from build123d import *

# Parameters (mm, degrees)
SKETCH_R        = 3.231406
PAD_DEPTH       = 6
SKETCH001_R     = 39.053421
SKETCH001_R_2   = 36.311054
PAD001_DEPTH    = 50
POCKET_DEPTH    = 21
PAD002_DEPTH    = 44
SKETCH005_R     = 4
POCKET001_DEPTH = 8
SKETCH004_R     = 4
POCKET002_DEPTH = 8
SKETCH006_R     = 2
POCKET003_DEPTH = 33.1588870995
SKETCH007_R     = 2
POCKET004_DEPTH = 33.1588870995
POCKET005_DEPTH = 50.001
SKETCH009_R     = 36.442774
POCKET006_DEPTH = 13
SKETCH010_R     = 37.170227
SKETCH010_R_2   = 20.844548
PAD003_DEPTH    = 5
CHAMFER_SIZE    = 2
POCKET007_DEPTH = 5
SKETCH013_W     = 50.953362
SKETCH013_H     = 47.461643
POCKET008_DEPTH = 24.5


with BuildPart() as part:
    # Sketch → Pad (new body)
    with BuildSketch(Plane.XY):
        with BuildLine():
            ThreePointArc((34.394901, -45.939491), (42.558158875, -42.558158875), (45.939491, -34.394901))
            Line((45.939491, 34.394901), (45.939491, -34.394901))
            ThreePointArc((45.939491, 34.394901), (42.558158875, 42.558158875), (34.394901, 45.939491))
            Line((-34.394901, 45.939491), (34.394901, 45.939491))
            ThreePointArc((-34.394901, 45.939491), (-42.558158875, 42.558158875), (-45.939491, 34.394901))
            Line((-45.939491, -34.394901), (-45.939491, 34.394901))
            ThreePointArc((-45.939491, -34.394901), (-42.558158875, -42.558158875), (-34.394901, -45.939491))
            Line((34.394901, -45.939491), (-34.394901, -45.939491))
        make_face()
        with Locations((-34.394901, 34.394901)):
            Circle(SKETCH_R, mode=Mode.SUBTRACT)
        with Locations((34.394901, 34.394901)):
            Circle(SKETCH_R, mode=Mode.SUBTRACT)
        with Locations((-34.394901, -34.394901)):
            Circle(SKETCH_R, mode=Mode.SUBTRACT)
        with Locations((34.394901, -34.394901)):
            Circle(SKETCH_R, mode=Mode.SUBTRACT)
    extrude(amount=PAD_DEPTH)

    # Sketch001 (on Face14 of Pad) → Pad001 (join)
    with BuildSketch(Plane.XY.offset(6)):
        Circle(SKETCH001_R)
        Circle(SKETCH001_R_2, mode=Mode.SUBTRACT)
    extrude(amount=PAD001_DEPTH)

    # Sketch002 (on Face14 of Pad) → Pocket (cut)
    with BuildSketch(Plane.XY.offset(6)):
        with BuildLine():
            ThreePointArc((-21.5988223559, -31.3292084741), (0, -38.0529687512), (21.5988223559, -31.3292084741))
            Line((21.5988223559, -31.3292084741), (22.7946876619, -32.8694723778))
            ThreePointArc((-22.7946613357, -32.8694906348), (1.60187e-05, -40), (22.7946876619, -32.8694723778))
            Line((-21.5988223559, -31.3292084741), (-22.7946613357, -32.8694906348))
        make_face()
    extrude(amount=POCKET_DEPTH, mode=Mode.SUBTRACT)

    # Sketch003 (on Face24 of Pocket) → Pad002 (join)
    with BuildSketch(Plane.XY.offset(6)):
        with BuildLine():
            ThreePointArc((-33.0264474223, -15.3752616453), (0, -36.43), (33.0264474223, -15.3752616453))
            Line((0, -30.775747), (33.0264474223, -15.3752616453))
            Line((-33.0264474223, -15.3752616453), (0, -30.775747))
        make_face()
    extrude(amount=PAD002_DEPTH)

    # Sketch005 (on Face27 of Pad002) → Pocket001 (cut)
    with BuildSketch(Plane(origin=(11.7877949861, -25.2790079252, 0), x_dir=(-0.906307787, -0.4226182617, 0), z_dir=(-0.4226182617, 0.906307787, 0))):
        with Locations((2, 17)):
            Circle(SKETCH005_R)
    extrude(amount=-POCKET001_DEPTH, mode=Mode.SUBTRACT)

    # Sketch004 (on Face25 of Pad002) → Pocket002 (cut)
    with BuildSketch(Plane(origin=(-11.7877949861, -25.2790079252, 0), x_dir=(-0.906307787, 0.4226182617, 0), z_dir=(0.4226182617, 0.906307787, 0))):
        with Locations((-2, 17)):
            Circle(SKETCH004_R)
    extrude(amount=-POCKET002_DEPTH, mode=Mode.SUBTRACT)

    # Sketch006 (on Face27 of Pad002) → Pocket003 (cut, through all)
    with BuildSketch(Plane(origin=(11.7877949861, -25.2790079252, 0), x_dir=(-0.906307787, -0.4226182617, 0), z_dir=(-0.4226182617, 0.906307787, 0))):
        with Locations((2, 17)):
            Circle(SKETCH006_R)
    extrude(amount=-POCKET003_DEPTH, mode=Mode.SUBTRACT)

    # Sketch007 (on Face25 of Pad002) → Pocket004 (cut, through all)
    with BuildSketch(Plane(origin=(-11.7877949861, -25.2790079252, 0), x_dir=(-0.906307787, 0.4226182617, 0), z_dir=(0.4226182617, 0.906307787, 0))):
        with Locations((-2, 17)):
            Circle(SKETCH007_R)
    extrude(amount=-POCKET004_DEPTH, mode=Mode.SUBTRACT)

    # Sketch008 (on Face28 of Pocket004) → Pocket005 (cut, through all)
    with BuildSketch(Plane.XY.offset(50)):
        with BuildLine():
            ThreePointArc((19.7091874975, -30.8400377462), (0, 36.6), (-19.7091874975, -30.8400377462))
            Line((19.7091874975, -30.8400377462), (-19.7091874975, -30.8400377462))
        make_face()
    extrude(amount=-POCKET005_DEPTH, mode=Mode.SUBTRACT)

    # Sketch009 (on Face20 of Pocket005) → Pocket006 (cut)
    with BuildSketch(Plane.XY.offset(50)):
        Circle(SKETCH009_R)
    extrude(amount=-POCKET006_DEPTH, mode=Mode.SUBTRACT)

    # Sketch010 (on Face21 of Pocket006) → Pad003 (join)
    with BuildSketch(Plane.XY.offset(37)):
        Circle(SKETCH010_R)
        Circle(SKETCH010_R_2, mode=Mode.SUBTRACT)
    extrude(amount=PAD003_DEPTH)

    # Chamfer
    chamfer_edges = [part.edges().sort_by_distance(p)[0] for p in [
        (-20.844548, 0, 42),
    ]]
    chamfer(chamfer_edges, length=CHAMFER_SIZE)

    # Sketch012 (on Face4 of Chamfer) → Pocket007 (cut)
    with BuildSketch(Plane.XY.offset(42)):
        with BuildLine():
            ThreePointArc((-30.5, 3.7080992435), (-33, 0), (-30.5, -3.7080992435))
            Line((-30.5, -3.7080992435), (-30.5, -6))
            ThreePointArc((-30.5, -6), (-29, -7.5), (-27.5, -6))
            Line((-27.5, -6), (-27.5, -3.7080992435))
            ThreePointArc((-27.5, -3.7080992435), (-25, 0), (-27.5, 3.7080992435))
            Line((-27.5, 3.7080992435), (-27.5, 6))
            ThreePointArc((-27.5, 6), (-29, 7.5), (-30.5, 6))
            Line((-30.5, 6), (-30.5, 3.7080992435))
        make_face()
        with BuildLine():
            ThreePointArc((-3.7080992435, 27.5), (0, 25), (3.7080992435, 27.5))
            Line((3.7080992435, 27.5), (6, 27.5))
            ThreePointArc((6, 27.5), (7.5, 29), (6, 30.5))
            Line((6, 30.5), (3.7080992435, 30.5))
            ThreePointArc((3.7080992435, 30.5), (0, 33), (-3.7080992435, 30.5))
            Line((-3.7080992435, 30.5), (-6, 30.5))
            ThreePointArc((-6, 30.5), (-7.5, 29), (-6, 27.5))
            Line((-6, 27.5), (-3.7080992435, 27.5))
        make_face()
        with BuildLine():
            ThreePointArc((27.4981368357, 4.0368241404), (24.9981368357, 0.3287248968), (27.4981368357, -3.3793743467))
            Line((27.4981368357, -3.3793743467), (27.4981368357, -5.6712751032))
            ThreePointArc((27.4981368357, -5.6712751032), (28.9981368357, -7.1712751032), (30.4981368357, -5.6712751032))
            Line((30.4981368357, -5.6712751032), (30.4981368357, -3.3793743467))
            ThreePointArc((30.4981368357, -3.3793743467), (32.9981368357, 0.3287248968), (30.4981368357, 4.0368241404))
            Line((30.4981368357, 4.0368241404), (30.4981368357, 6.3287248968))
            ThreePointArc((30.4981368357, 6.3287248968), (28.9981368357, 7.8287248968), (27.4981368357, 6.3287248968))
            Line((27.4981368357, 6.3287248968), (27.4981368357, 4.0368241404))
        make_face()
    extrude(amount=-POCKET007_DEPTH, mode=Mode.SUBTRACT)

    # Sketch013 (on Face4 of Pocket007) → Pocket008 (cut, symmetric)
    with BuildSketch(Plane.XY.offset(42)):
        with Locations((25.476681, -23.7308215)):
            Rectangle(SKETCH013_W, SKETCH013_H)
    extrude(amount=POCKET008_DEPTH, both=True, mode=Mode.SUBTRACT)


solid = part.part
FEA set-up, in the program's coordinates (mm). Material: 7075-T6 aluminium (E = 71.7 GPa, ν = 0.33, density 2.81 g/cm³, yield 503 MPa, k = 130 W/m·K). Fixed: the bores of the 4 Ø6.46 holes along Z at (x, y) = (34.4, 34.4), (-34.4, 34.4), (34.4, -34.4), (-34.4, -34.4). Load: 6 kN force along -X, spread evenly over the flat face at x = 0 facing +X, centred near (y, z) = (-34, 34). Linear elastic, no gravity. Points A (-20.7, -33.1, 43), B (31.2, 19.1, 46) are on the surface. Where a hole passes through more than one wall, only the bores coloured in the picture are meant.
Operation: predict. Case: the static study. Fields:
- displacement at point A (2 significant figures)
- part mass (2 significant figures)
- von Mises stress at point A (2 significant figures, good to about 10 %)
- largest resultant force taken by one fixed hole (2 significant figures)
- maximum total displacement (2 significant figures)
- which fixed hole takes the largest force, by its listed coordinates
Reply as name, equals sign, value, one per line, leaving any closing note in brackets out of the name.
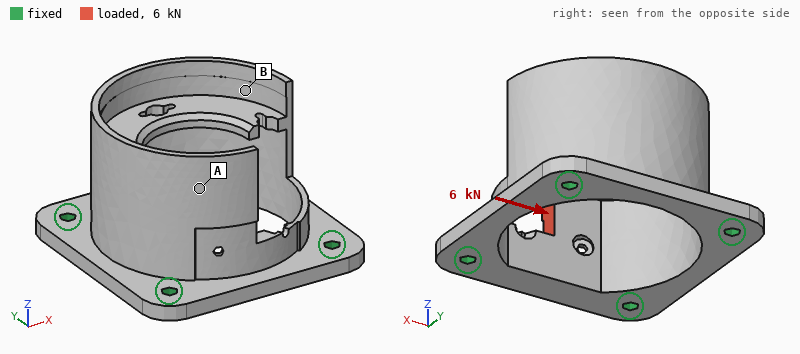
displacement at point A = 0.25 mm
part mass = 170 g
von Mises stress at point A = 54 MPa
largest resultant force taken by one fixed hole = 4.6 kN
maximum total displacement = 0.47 mm
which fixed hole takes the largest force, by its listed coordinates = (34.4, -34.4)
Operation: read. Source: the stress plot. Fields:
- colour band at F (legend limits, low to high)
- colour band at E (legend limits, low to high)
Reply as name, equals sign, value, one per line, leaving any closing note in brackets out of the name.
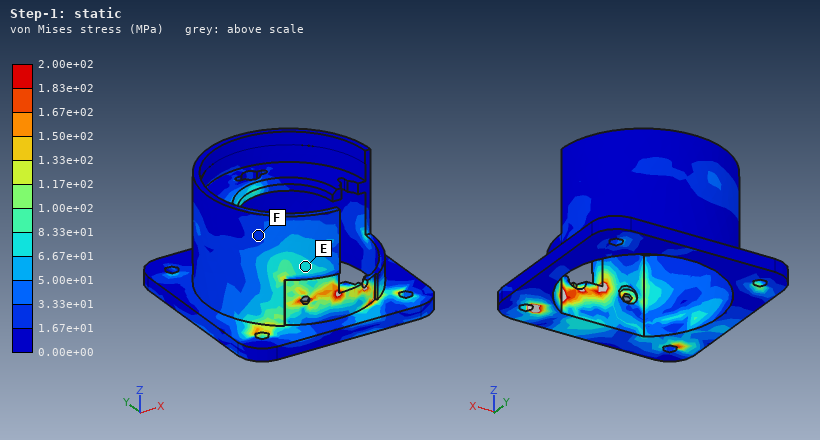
colour band at F = 1.67e+01 to 3.33e+01 MPa
colour band at E = 6.67e+01 to 8.33e+01 MPa
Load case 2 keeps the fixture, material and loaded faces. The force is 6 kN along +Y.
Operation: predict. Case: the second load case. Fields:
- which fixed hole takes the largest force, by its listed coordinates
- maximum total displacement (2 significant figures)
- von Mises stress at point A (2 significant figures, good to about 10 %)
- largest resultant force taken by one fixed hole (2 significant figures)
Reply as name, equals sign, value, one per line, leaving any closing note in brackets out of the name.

which fixed hole takes the largest force, by its listed coordinates = (-34.4, -34.4)
maximum total displacement = 1.0 mm
von Mises stress at point A = 63 MPa
largest resultant force taken by one fixed hole = 4.8 kN
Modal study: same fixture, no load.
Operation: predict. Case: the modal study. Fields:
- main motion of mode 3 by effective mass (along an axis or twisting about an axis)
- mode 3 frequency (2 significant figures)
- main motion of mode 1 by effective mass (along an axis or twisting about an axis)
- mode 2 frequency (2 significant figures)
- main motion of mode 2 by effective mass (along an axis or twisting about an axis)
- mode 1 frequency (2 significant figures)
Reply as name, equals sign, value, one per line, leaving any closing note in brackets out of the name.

main motion of mode 3 by effective mass = along X
mode 3 frequency = 5000 Hz
main motion of mode 1 by effective mass = along X
mode 2 frequency = 3600 Hz
main motion of mode 2 by effective mass = along Y
mode 1 frequency = 3300 Hz
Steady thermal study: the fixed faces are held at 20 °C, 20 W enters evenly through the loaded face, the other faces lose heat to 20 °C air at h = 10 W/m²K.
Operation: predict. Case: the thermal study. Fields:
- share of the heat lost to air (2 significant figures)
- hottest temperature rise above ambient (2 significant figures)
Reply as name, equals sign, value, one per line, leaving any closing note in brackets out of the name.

share of the heat lost to air = 10 %
hottest temperature rise above ambient = 30 K
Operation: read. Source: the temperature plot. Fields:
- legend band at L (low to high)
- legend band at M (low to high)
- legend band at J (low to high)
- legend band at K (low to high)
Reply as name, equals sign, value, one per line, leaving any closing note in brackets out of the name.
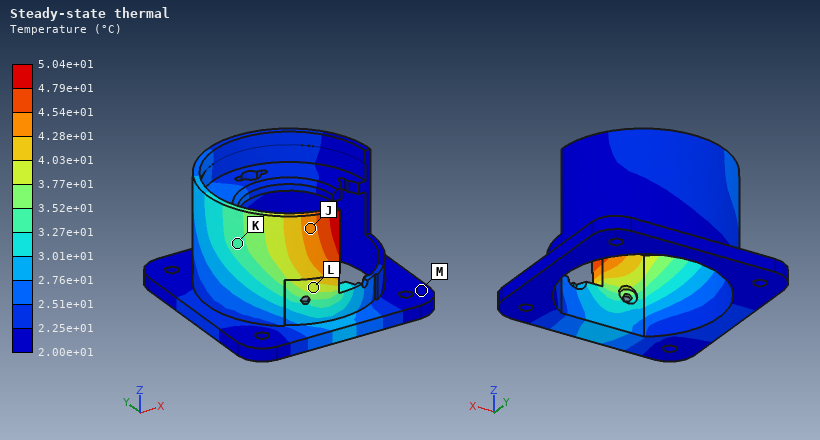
legend band at L = 3.77e+01 to 4.03e+01 °C
legend band at M = 2.00e+01 to 2.25e+01 °C
legend band at J = 4.28e+01 to 4.54e+01 °C
legend band at K = 3.27e+01 to 3.52e+01 °C
